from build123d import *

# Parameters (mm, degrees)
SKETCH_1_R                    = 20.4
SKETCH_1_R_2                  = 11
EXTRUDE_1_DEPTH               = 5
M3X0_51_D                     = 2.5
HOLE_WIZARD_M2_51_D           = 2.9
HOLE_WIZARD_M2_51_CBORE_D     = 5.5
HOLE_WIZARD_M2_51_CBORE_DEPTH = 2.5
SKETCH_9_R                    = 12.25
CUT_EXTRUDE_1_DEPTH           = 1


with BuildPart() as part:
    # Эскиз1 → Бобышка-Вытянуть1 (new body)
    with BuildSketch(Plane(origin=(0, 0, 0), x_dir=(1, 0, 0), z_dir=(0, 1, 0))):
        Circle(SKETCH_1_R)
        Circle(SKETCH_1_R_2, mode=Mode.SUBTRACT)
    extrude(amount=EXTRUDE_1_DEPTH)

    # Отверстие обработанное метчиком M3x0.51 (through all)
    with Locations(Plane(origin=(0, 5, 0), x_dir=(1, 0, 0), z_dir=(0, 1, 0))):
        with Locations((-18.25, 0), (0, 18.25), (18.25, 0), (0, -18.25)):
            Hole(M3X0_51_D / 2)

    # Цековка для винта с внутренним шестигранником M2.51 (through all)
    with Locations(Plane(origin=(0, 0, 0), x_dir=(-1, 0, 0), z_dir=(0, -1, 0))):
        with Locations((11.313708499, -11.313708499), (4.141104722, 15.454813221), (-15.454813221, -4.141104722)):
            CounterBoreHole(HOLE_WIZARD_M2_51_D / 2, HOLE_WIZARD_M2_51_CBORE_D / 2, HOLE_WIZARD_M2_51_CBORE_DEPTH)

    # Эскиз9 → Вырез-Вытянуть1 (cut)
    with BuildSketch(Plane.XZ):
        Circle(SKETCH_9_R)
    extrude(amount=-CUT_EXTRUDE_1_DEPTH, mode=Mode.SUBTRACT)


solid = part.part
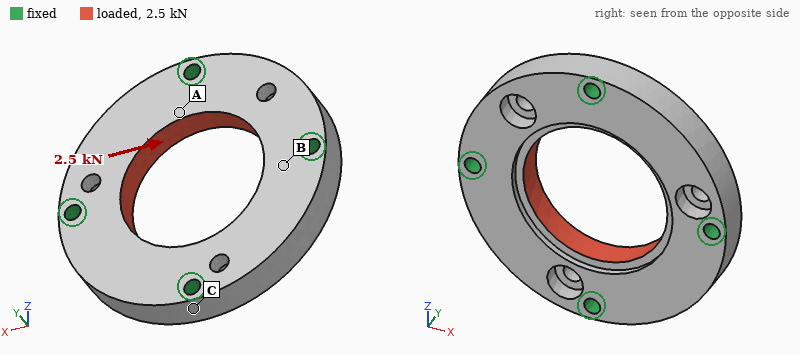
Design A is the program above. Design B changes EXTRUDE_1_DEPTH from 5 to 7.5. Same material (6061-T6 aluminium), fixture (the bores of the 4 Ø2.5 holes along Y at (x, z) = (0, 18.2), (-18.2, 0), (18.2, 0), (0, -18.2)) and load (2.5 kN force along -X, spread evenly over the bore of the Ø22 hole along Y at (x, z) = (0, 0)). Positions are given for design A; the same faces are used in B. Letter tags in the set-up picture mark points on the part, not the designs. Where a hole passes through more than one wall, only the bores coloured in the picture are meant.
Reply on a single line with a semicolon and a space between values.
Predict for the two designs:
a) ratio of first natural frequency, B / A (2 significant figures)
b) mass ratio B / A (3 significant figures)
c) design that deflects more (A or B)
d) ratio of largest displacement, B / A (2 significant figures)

1.3; 1.53; A; 0.64
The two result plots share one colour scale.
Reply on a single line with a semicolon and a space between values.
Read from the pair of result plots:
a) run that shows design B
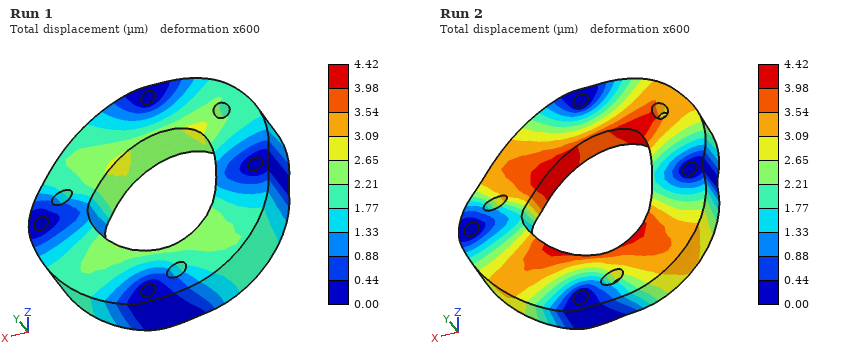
Run 1
